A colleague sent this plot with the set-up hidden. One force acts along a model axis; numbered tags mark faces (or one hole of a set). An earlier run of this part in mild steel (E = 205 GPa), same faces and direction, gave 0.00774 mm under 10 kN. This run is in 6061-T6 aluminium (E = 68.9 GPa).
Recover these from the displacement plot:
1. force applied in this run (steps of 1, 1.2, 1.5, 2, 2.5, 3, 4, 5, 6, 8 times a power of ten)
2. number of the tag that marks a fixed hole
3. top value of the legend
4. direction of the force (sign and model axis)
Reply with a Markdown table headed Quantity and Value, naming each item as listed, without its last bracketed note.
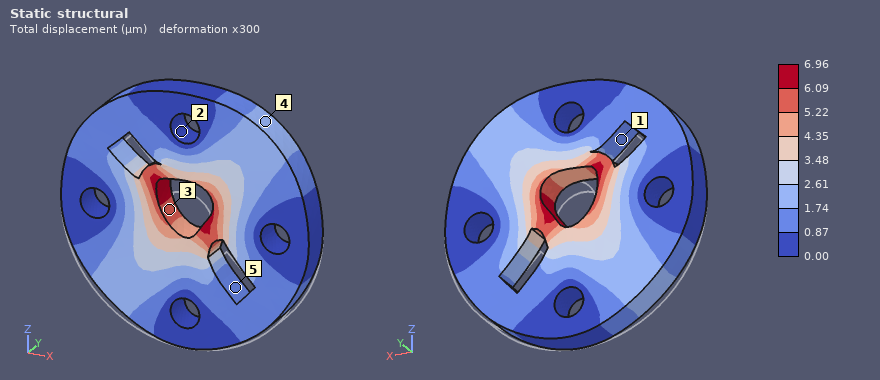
| Quantity | Value |
|---|---|
| force applied in this run | 3 kN |
| number of the tag that marks a fixed hole | 2 |
| top value of the legend | 6.96 µm |
| direction of the force | +Z |
